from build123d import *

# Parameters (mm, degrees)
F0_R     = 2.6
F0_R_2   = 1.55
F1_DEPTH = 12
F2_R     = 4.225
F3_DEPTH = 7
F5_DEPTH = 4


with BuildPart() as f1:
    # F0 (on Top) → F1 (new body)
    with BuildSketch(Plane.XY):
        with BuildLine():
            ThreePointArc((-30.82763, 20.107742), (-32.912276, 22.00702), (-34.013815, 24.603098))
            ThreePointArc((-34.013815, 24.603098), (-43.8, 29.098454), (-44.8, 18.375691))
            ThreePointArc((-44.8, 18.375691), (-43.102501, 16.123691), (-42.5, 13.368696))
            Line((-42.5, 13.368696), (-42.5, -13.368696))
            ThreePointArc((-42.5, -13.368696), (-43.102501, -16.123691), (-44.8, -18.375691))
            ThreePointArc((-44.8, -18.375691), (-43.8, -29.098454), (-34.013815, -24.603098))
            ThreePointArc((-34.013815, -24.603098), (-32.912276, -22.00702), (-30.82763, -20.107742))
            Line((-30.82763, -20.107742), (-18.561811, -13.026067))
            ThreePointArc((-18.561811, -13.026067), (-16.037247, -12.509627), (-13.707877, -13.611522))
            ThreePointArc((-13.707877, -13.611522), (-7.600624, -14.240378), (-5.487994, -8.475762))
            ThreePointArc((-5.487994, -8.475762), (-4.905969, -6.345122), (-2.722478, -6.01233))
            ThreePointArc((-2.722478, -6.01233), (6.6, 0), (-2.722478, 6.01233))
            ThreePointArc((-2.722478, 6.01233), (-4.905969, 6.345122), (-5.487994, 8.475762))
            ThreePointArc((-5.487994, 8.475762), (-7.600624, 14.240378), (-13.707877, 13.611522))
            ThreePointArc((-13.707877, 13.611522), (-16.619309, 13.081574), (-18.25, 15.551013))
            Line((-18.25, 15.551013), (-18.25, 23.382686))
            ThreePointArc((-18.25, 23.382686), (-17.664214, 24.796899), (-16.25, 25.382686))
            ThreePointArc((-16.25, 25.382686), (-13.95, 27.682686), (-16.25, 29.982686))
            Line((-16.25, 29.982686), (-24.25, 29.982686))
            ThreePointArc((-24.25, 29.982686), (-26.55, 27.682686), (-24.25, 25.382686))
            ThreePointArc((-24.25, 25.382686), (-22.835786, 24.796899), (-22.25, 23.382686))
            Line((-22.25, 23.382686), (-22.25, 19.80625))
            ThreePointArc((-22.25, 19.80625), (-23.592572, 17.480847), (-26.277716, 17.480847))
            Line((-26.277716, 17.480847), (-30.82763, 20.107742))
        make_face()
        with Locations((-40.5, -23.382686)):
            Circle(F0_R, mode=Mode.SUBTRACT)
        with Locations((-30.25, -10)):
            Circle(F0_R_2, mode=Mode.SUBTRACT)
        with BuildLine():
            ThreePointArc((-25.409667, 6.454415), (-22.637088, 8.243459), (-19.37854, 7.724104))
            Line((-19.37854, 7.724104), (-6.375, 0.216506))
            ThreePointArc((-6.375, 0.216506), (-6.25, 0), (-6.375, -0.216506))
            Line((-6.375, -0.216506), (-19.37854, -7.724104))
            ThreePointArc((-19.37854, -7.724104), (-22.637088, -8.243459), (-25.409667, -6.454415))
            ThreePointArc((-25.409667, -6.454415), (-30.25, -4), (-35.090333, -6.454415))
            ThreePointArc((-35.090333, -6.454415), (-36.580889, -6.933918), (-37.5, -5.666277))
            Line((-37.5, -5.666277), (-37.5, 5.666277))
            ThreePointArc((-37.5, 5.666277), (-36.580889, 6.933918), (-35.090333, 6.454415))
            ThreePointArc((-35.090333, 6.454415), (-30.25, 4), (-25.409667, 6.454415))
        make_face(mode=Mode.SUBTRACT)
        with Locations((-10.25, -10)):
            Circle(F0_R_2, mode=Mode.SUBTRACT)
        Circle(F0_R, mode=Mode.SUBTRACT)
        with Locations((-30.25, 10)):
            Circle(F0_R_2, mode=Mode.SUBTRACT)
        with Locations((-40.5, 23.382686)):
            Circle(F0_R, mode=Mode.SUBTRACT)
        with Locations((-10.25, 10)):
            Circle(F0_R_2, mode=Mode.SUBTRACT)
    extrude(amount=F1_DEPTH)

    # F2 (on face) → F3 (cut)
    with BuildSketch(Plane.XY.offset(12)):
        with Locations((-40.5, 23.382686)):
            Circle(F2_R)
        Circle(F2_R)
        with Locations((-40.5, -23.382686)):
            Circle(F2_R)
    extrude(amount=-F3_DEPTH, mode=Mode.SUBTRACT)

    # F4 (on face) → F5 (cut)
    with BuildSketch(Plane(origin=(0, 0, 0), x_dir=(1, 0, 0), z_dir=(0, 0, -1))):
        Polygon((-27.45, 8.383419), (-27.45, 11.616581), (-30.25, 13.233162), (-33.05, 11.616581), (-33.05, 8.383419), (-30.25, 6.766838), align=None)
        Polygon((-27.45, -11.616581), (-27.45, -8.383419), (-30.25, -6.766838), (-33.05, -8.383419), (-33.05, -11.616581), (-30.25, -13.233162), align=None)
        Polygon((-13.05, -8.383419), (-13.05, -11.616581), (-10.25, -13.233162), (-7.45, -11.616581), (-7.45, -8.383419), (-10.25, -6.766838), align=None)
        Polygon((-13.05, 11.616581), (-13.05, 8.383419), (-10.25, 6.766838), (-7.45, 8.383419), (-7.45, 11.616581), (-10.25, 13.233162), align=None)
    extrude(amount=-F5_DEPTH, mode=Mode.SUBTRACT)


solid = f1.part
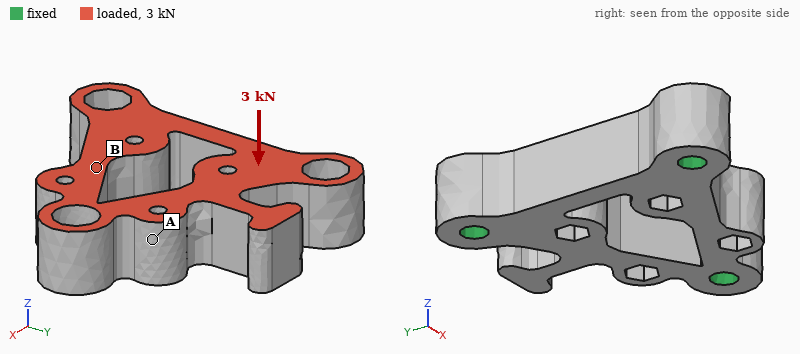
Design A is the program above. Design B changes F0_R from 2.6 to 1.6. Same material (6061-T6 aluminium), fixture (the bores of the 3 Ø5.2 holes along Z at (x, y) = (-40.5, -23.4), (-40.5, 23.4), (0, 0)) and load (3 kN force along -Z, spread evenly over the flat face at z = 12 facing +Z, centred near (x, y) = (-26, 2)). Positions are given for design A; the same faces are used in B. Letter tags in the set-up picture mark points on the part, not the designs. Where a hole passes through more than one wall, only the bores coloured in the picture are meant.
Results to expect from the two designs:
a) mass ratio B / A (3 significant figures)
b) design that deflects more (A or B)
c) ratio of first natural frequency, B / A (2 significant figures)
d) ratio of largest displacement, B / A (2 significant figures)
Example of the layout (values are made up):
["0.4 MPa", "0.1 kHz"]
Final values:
["1.01", "B", "0.99", "1.1"]
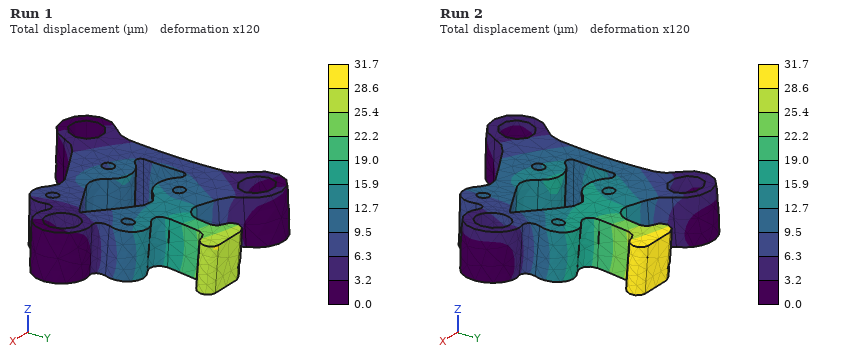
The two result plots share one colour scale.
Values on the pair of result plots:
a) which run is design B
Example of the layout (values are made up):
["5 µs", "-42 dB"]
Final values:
["Run 2"]
